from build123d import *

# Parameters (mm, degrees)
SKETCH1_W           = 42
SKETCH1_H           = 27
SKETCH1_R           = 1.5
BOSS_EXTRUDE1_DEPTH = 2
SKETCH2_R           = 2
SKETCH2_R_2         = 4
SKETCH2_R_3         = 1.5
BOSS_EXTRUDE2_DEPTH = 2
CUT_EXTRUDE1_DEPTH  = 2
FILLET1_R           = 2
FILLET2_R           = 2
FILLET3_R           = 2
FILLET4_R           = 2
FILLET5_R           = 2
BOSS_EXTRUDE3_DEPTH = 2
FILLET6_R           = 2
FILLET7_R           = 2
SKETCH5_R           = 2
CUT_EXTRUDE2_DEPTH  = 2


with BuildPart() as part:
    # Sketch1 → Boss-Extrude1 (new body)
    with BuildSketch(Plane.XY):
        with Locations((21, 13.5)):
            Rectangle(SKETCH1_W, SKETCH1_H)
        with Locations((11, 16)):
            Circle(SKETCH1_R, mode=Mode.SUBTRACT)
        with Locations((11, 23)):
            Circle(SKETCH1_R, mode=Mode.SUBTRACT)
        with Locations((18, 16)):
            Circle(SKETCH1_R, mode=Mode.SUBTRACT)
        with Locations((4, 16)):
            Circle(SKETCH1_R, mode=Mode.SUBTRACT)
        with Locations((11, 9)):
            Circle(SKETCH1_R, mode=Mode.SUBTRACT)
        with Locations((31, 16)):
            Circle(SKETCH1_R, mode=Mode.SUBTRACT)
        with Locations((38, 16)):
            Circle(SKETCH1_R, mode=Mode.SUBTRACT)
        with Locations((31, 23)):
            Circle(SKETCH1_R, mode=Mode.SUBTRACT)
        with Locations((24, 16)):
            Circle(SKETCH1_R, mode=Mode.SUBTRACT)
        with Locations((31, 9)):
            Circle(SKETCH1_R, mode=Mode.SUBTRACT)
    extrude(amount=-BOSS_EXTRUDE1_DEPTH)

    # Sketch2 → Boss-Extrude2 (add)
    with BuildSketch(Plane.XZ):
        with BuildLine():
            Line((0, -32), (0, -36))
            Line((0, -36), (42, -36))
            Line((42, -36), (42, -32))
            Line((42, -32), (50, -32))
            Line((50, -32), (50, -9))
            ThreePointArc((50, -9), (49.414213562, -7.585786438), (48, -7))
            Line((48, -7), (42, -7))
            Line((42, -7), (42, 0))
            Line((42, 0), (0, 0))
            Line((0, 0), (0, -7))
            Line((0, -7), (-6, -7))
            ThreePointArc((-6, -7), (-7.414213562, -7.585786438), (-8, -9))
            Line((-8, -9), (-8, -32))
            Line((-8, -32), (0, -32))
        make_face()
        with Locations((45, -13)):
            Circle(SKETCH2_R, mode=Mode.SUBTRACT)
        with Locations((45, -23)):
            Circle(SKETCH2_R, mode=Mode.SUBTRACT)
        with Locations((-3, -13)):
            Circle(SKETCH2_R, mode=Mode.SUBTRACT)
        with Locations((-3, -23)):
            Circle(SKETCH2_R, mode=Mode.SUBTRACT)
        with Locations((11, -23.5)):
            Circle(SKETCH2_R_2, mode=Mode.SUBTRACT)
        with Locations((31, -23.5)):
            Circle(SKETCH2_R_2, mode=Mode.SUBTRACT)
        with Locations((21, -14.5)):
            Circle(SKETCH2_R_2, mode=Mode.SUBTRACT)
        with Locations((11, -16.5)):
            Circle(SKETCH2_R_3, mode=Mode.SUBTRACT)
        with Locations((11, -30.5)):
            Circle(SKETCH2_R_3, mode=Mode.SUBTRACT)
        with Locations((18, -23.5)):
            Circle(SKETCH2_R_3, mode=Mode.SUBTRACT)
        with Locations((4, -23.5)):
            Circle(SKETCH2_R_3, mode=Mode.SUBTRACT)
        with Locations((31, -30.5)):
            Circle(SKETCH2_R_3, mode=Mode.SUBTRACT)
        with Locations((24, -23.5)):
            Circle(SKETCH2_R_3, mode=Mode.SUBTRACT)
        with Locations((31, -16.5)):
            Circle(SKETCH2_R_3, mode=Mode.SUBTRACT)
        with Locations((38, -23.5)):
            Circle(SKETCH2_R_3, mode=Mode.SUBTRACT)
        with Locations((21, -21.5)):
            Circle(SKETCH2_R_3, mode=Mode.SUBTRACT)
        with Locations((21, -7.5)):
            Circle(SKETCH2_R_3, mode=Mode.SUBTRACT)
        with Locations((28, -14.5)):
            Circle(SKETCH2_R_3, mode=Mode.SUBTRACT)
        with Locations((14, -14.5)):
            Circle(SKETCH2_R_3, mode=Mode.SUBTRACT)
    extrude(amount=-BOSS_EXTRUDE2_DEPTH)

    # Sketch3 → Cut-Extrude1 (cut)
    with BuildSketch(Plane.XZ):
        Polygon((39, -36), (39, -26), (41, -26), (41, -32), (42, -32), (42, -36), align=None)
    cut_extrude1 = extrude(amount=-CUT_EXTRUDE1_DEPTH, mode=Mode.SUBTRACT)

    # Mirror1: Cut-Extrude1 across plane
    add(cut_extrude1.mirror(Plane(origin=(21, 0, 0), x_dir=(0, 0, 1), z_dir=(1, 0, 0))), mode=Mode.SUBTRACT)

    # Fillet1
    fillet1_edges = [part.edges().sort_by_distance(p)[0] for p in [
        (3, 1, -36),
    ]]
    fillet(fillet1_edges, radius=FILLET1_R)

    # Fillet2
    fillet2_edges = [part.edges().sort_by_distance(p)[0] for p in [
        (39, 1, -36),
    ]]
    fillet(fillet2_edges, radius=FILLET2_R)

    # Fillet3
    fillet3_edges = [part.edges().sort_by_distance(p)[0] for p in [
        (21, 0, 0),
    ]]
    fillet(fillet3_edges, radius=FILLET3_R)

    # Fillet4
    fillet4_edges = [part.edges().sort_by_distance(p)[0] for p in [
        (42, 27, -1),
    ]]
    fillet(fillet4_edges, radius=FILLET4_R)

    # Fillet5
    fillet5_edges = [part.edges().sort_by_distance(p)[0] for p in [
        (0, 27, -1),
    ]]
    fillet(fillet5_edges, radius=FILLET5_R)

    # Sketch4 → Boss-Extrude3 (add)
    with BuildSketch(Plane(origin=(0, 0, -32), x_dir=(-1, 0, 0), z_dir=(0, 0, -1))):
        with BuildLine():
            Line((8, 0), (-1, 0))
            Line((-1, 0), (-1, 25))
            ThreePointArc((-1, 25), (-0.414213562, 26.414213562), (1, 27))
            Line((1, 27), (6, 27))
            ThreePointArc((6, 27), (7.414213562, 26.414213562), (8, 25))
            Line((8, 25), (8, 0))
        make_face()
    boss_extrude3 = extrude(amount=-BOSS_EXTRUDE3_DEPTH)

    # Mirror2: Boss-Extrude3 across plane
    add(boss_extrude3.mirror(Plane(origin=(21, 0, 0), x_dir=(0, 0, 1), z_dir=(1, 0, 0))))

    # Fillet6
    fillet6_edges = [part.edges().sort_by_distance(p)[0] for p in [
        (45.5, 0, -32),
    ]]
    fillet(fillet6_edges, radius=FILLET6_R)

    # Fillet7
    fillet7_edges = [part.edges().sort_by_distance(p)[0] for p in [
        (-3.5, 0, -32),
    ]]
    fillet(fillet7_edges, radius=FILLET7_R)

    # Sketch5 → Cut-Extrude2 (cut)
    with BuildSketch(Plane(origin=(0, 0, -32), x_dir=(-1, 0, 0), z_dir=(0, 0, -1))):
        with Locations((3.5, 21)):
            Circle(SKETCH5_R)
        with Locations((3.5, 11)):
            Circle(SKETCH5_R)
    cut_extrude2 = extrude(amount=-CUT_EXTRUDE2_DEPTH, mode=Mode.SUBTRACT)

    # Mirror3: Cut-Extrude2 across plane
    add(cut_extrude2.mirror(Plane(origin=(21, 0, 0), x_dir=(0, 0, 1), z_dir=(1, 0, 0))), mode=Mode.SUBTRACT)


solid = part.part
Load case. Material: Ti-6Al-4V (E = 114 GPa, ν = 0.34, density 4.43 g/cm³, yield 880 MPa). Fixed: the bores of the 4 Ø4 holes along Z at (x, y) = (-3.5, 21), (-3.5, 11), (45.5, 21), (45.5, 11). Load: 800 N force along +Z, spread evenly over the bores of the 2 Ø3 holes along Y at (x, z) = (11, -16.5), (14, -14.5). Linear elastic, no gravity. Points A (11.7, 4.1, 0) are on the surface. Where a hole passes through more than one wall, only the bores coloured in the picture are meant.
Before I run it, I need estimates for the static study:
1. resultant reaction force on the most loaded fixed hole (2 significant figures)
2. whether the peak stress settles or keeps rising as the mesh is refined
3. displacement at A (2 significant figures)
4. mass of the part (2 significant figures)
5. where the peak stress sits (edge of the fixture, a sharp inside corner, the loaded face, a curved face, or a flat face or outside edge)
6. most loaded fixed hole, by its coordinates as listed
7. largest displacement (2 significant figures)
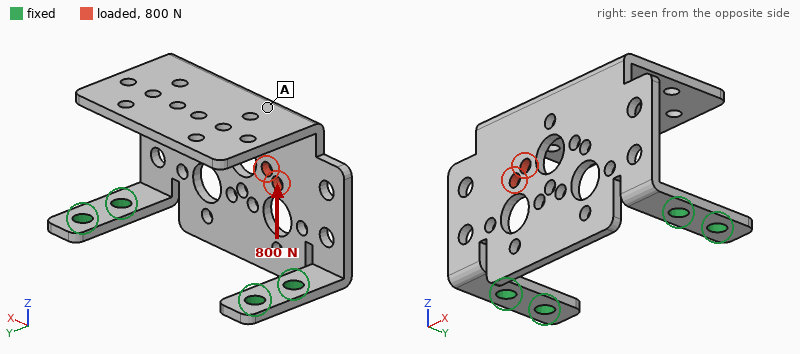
550 N
keeps rising
0.67 mm
26 g
edge of the fixture
(-3.5, 11)
0.80 mm
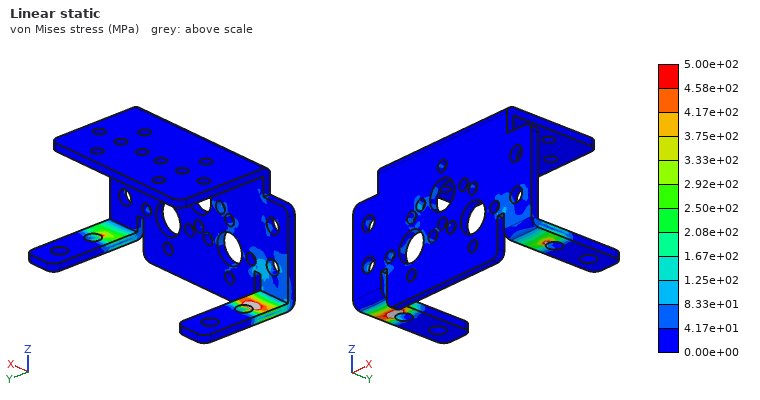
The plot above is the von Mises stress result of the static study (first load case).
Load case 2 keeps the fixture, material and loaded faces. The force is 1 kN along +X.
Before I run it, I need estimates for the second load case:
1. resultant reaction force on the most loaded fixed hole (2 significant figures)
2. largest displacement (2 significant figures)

710 N
0.28 mm
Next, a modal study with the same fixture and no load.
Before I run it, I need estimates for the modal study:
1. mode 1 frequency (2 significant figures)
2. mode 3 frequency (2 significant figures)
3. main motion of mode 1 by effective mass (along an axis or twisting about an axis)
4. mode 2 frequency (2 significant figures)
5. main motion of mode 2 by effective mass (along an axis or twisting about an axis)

380 Hz
1500 Hz
along Y
1100 Hz
along X
